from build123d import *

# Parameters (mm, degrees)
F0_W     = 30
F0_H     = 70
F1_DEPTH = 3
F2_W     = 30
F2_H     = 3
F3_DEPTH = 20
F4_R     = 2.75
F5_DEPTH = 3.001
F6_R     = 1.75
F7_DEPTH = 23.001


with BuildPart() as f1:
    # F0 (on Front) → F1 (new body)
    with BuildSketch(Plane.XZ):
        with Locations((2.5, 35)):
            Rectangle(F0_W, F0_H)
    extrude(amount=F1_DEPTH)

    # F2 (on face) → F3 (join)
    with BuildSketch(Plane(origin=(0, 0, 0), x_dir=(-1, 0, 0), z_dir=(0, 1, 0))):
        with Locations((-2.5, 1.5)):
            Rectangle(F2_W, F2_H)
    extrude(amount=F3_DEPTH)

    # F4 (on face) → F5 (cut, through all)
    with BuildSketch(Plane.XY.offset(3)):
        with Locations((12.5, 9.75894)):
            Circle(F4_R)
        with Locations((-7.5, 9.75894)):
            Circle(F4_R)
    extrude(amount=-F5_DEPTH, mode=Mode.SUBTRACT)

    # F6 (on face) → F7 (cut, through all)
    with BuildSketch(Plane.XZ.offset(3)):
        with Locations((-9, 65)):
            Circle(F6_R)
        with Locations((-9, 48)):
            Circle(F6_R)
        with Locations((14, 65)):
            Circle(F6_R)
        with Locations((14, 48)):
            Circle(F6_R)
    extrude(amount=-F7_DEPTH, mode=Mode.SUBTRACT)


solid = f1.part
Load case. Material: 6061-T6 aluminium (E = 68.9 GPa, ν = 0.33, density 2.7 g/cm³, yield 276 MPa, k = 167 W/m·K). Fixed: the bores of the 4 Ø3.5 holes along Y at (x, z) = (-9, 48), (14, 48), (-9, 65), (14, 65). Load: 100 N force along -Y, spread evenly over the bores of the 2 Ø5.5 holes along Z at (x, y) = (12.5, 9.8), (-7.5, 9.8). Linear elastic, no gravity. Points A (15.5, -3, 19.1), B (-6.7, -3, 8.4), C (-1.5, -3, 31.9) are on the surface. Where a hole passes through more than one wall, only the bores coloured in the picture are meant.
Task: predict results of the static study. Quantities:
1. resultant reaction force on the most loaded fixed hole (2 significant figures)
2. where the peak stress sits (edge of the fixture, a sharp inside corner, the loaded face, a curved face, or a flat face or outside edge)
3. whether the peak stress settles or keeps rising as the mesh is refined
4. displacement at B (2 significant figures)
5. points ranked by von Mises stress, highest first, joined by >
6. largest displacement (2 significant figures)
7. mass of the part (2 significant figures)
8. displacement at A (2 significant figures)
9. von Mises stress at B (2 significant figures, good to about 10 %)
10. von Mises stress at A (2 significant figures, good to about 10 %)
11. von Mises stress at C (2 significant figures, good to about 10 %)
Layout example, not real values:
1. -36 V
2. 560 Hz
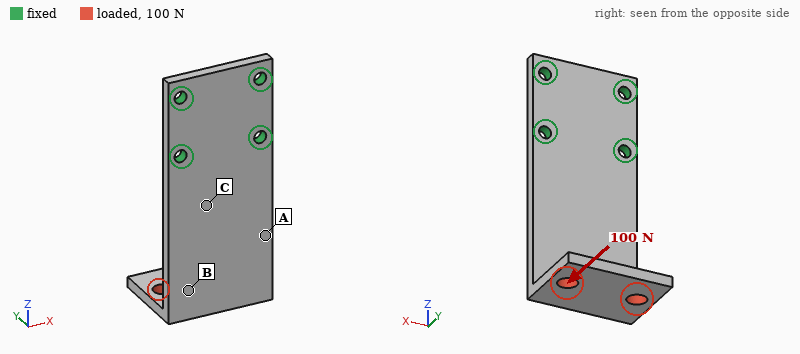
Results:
1. 86 N
2. edge of the fixture
3. keeps rising
4. 0.55 mm
5. C > A > B
6. 0.89 mm
7. 21 g
8. 0.32 mm
9. 17 MPa
10. 41 MPa
11. 64 MPa
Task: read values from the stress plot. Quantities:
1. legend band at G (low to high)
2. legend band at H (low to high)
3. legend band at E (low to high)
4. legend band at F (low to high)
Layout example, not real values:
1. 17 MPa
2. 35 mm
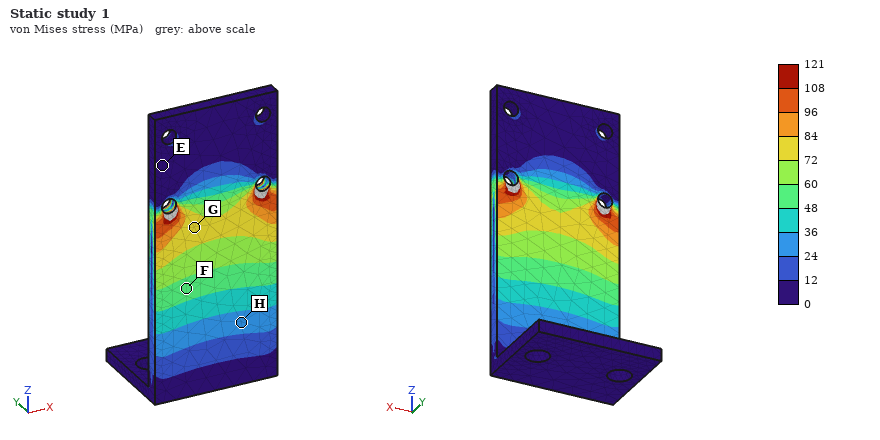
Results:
1. 72 to 84 MPa
2. 24 to 36 MPa
3. 0 to 12 MPa
4. 48 to 60 MPa
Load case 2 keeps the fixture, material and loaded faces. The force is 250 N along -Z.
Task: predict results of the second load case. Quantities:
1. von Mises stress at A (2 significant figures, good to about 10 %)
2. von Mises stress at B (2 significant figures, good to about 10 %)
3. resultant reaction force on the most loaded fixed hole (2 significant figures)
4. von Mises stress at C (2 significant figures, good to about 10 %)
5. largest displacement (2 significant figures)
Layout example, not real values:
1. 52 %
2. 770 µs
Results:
1. 61 MPa
2. 57 MPa
3. 110 N
4. 57 MPa
5. 0.94 mm
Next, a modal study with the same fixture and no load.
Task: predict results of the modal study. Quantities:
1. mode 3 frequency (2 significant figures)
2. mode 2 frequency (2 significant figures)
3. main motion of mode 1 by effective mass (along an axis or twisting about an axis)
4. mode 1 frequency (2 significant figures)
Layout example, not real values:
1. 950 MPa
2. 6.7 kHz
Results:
1. 2900 Hz
2. 1800 Hz
3. along Y
4. 650 Hz
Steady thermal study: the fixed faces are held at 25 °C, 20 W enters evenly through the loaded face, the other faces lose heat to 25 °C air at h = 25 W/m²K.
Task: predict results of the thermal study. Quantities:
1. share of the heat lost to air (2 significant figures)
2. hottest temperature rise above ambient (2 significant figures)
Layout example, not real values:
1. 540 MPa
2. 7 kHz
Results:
1. 21 %
2. 69 K
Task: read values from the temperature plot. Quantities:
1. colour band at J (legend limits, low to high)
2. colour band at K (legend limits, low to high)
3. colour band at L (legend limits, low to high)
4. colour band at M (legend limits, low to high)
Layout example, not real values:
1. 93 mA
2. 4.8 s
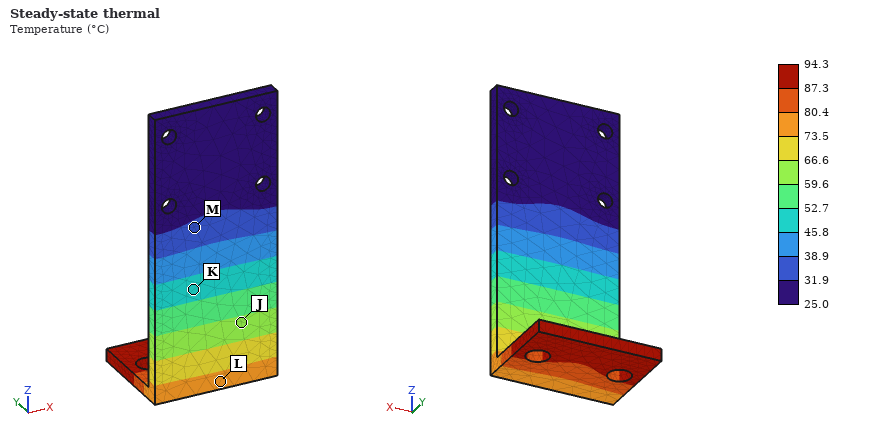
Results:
1. 59.6 to 66.6 °C
2. 45.8 to 52.7 °C
3. 73.5 to 80.4 °C
4. 31.9 to 38.9 °C
